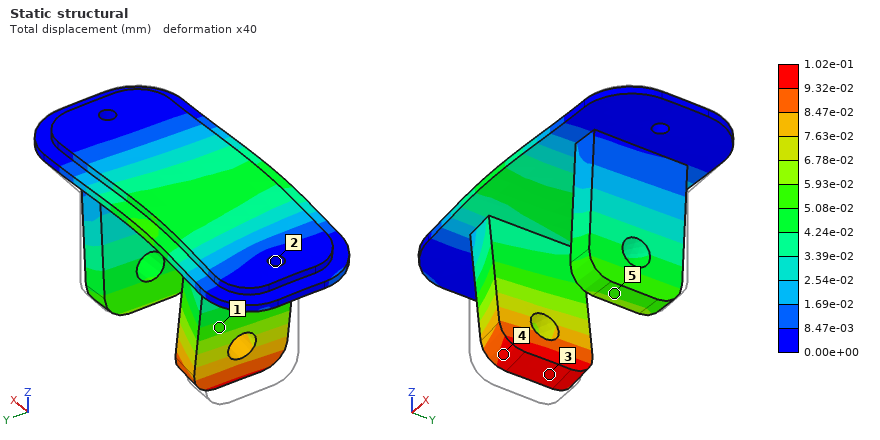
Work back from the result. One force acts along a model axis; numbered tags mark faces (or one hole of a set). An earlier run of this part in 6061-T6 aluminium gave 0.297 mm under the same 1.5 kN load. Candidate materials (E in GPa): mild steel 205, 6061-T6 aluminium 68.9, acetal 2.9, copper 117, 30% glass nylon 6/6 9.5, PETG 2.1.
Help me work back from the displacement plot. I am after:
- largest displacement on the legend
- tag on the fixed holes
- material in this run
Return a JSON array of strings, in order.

["1.02e-01 mm", "2", "mild steel"]
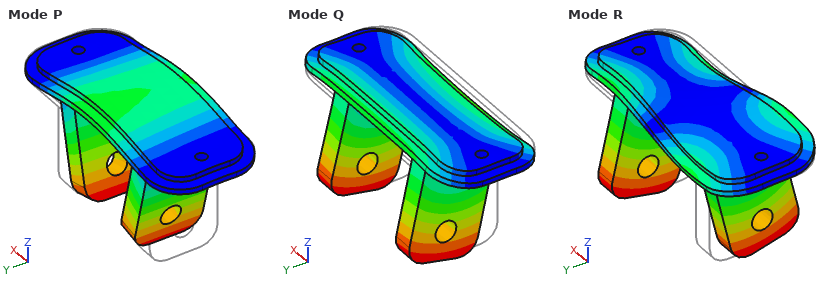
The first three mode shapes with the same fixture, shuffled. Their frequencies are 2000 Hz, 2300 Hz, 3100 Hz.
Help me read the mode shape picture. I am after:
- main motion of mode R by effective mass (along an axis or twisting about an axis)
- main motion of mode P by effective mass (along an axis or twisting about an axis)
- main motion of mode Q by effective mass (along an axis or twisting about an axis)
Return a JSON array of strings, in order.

["twisting about Z", "along Z", "along Y"]
